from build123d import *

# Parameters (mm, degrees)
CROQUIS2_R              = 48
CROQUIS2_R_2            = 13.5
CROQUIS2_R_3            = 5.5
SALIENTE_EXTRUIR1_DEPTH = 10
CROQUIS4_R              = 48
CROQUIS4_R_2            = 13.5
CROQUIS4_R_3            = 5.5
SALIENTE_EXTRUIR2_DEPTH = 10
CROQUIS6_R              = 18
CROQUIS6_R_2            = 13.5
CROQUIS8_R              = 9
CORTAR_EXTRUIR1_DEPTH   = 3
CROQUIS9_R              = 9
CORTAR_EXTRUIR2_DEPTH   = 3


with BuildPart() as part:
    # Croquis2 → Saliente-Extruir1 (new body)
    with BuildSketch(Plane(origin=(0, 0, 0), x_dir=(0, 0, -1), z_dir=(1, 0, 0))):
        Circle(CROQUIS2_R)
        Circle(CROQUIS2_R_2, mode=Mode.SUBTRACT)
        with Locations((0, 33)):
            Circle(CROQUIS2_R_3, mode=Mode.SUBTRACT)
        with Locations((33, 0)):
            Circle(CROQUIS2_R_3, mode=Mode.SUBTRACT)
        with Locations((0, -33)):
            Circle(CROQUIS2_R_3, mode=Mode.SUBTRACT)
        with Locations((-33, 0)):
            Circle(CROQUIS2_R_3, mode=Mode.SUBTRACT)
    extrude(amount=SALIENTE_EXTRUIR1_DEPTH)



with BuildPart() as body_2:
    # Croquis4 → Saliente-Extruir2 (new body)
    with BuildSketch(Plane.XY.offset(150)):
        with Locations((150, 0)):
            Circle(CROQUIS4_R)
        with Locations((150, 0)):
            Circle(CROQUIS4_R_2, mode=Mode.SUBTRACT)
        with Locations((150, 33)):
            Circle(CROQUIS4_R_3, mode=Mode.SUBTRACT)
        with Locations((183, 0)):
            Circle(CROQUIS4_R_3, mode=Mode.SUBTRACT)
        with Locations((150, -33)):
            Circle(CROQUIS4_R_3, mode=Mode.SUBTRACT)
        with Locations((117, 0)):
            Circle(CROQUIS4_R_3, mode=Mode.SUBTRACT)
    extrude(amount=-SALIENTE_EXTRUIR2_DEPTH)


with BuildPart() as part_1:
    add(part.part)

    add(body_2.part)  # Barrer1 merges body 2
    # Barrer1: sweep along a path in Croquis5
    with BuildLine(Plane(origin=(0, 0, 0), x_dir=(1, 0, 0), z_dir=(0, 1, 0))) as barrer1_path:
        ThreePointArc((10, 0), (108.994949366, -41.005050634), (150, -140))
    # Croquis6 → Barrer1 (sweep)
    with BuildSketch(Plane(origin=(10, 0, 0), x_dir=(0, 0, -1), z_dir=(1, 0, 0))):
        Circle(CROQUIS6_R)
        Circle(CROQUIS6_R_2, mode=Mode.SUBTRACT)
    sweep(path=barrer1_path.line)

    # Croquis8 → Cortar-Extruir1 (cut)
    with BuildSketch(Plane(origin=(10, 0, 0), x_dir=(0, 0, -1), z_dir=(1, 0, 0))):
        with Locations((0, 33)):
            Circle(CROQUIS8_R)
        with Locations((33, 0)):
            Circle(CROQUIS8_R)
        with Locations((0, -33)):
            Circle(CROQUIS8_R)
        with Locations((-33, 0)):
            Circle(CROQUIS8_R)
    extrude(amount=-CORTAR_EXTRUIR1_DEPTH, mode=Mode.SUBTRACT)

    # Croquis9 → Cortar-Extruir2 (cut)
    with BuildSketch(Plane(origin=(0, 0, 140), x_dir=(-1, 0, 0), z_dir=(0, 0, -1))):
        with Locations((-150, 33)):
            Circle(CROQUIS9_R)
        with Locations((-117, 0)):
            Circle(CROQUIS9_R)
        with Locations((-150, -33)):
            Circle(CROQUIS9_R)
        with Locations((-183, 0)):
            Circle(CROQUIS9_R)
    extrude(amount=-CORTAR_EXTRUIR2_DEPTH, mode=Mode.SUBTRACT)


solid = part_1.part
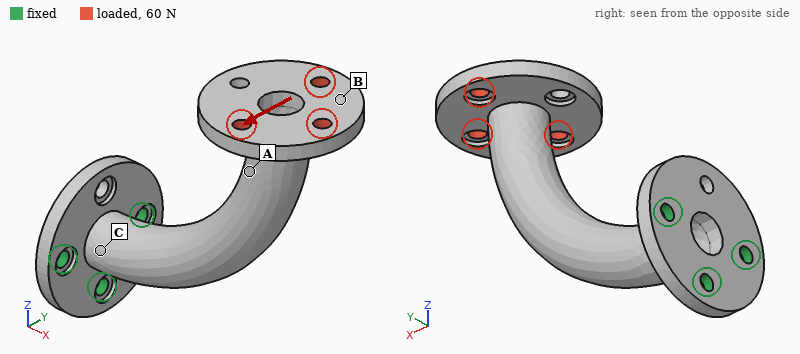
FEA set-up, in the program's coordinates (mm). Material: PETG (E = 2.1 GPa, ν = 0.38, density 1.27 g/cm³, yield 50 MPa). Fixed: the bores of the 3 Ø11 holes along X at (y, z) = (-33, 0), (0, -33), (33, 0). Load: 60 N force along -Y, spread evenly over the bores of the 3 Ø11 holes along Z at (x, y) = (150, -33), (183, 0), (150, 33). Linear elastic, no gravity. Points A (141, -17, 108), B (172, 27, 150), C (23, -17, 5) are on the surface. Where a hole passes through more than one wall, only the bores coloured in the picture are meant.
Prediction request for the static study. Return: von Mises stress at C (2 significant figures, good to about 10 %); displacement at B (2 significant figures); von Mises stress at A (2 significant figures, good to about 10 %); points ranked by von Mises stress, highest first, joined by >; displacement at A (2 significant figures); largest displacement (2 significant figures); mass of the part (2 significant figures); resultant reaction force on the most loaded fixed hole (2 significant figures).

3.3 MPa
2.7 mm
0.84 MPa
C > A > B
1.9 mm
2.9 mm
280 g
210 N
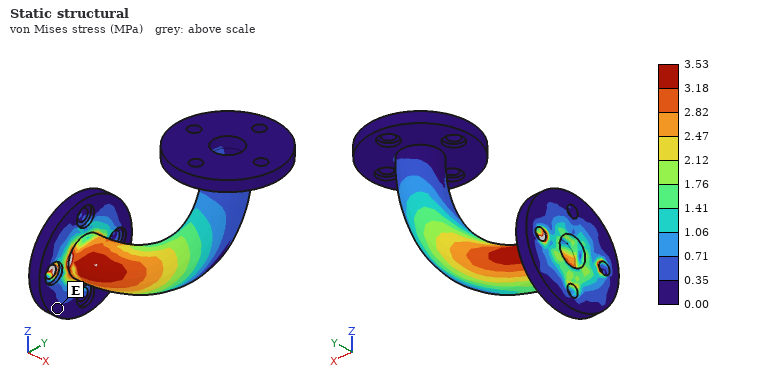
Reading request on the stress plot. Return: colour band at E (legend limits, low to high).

0.00 to 0.35 MPa
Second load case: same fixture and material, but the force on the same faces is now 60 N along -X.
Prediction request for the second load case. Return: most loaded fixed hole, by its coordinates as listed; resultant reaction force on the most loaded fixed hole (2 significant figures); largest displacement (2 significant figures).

(0, -33)
220 N
3.0 mm
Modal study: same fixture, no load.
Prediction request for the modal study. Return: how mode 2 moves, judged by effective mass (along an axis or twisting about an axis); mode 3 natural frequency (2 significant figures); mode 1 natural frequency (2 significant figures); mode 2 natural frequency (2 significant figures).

along Y
280 Hz
67 Hz
77 Hz
